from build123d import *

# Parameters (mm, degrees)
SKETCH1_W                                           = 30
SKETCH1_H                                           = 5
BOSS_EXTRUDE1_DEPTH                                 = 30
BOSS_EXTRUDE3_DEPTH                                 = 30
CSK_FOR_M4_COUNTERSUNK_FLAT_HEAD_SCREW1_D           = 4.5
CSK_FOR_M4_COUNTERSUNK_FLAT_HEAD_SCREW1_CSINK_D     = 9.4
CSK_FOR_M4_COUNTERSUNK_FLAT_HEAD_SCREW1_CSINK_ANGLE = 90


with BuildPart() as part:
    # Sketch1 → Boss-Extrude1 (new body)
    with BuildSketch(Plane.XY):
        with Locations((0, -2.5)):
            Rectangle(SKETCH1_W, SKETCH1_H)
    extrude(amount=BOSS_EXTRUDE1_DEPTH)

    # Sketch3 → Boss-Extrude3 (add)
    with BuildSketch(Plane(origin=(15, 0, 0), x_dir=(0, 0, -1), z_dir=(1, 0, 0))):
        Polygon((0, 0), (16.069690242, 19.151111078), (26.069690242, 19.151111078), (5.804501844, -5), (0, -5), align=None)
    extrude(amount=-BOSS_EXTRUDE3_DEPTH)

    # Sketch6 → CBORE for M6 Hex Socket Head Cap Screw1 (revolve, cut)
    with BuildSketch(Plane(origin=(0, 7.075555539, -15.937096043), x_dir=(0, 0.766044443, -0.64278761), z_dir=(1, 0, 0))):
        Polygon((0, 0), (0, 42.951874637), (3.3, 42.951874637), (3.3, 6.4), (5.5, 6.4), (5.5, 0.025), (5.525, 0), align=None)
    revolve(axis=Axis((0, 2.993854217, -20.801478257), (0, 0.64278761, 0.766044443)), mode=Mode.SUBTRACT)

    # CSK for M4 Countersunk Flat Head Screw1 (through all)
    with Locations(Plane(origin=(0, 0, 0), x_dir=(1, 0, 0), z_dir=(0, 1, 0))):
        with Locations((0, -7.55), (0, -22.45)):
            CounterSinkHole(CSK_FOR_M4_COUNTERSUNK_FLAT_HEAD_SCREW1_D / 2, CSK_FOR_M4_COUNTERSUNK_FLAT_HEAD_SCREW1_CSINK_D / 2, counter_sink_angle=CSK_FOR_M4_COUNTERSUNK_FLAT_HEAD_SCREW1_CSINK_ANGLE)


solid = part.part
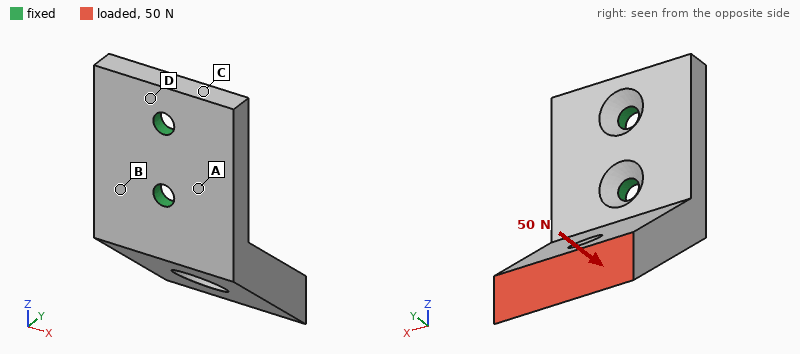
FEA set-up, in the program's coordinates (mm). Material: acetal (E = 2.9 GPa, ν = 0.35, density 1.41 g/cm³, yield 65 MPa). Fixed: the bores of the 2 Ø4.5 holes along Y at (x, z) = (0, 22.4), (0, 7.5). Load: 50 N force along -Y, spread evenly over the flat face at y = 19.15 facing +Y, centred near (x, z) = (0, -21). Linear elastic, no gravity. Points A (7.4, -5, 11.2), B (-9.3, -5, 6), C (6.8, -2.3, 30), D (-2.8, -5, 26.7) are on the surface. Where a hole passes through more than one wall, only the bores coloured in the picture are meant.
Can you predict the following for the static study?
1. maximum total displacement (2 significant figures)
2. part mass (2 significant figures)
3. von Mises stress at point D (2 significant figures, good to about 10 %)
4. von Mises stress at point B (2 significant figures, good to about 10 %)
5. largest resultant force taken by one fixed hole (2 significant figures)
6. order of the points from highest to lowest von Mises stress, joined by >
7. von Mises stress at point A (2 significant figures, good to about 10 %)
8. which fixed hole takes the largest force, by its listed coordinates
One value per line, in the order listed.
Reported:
0.80 mm
15 g
2.3 MPa
7.9 MPa
130 N
B > A > D > C
4.5 MPa
(0, 7.5)
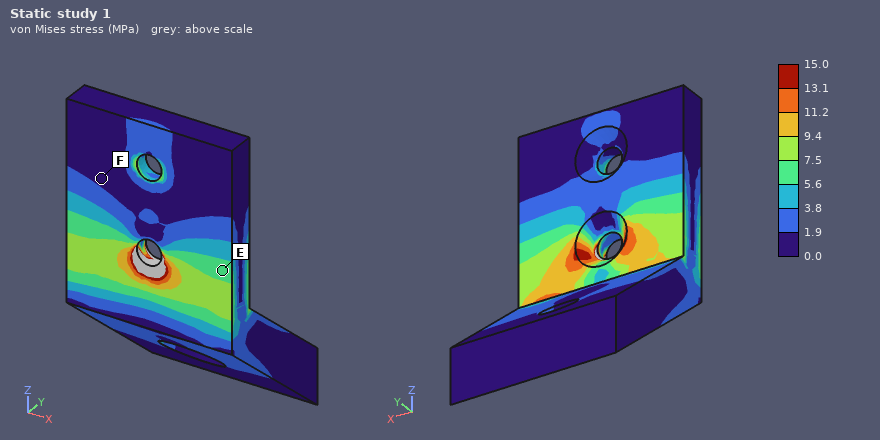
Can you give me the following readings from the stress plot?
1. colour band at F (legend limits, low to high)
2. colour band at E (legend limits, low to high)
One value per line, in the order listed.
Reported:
0.0 to 1.9 MPa
5.6 to 7.5 MPa
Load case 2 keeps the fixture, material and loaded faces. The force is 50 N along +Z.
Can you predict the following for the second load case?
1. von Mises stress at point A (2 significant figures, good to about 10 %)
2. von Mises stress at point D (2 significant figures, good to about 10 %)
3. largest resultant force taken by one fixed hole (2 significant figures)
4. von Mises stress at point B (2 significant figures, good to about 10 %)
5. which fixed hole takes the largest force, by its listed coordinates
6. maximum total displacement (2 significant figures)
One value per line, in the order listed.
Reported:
3.4 MPa
2.2 MPa
80 N
6.7 MPa
(0, 22.4)
0.72 mm
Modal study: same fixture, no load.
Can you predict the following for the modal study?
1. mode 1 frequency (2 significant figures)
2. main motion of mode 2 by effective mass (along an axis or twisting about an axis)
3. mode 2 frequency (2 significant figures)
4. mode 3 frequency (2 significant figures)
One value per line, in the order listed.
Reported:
640 Hz
along X
920 Hz
2500 Hz
